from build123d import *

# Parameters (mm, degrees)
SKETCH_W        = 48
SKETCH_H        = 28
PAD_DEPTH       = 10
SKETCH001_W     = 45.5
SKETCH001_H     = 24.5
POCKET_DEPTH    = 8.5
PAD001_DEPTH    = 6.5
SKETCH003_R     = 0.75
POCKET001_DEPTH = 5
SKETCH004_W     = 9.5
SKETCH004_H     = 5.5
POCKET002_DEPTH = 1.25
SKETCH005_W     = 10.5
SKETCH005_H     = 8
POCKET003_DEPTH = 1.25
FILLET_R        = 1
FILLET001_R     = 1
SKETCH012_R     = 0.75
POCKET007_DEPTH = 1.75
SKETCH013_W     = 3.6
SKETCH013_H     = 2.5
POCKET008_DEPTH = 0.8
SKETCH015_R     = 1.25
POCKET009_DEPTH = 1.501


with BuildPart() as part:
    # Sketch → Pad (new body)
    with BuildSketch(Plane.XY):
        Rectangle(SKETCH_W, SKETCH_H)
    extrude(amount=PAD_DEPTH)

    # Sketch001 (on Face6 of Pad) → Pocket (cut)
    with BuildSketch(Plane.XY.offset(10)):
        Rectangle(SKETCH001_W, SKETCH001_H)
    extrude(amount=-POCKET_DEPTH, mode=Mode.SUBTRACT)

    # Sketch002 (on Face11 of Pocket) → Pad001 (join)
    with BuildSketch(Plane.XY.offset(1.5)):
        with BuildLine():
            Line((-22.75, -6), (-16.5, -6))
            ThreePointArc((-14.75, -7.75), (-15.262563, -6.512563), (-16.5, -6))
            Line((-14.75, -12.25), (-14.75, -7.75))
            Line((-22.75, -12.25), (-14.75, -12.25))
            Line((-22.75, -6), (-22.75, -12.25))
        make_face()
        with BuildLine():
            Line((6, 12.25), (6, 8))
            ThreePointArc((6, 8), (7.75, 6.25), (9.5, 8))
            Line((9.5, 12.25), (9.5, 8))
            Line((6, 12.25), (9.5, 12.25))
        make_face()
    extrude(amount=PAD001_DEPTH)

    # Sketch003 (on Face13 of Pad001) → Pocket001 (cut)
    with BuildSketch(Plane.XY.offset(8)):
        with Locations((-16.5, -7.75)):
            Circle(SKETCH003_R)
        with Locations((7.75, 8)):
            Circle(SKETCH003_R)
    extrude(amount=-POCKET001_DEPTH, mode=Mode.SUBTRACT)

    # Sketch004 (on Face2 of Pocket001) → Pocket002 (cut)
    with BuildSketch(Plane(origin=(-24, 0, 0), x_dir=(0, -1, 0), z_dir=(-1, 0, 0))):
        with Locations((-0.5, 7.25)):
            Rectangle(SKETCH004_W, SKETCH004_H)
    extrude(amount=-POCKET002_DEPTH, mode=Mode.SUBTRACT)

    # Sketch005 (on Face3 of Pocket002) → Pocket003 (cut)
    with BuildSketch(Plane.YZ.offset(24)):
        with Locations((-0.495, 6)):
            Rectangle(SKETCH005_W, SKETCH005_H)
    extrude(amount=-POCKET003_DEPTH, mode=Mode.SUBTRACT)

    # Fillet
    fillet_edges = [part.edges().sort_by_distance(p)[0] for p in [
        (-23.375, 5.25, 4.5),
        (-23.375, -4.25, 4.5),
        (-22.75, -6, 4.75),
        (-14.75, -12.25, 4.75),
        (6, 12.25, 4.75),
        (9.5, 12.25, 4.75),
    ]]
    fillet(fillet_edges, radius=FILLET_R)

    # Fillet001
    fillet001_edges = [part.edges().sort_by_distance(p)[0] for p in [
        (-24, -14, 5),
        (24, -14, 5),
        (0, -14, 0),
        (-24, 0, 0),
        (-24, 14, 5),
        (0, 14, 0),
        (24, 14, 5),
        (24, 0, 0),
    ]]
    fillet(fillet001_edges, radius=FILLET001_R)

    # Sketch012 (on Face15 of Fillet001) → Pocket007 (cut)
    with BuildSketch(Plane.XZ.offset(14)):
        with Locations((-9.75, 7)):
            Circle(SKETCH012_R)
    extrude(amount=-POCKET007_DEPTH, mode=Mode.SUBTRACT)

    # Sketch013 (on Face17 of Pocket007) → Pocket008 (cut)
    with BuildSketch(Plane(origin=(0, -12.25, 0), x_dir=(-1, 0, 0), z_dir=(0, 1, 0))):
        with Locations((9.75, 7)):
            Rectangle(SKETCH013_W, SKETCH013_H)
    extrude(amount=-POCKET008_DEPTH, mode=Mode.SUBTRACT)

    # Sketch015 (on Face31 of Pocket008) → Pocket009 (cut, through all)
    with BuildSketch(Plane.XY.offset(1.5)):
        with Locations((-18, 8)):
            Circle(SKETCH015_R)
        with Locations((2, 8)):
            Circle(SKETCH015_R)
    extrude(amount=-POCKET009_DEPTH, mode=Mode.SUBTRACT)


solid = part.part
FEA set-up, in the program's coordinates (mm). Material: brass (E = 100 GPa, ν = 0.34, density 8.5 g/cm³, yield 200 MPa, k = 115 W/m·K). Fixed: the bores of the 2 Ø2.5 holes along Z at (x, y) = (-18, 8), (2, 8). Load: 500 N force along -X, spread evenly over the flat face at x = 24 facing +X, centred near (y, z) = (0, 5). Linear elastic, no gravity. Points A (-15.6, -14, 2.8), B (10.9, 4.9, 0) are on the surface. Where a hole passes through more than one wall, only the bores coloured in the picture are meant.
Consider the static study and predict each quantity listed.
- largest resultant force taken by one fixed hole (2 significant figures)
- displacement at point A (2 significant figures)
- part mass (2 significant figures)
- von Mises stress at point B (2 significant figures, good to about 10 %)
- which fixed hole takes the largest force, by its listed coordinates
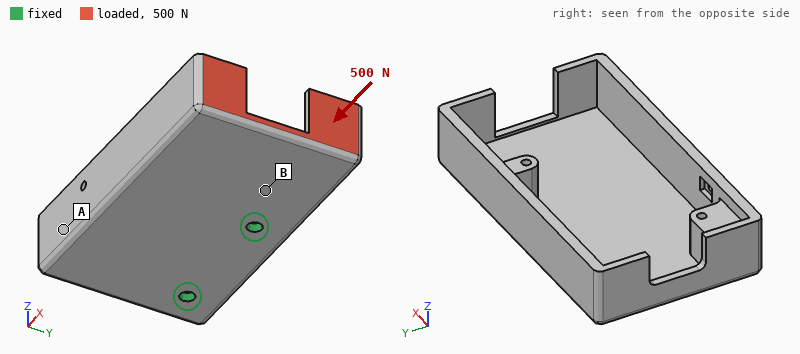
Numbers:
350 N
0.029 mm
35 g
22 MPa
(2, 8)
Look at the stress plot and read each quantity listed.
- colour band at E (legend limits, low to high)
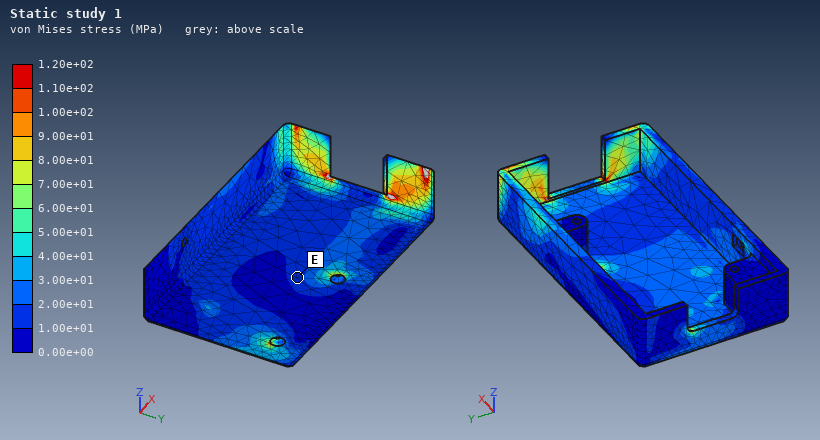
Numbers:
1.00e+01 to 2.00e+01 MPa
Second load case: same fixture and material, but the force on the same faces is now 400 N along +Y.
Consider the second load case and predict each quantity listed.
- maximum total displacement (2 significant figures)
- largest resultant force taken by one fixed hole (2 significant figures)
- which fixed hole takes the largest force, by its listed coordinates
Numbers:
0.36 mm
810 N
(2, 8)
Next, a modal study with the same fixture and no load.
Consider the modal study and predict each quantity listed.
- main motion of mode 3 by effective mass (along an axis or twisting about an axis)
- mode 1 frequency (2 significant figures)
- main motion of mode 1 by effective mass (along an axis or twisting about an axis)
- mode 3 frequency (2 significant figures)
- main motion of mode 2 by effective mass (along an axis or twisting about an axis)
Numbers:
along Z
1000 Hz
along Z
3800 Hz
twisting about Y
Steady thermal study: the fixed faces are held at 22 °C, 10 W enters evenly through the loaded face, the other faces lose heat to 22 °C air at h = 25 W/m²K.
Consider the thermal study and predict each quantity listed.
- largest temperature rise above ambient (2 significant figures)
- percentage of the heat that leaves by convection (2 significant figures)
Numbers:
45 K
18 %
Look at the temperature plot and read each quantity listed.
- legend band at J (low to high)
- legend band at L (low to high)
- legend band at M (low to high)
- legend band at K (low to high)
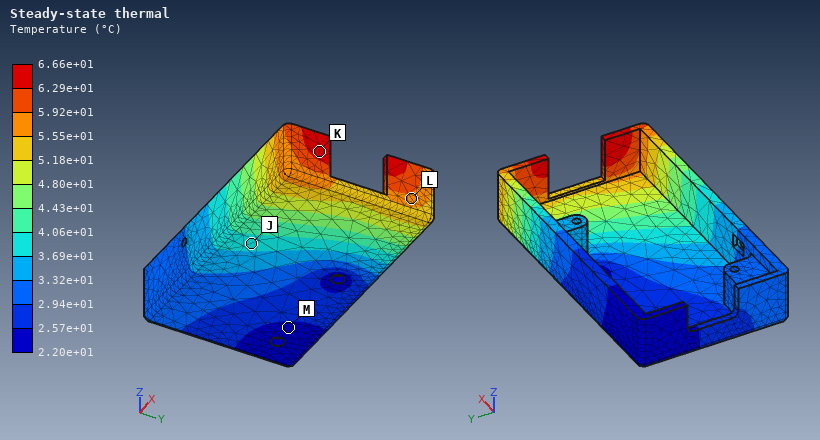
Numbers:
3.69e+01 to 4.06e+01 °C
5.55e+01 to 5.92e+01 °C
2.20e+01 to 2.57e+01 °C
6.29e+01 to 6.66e+01 °C
